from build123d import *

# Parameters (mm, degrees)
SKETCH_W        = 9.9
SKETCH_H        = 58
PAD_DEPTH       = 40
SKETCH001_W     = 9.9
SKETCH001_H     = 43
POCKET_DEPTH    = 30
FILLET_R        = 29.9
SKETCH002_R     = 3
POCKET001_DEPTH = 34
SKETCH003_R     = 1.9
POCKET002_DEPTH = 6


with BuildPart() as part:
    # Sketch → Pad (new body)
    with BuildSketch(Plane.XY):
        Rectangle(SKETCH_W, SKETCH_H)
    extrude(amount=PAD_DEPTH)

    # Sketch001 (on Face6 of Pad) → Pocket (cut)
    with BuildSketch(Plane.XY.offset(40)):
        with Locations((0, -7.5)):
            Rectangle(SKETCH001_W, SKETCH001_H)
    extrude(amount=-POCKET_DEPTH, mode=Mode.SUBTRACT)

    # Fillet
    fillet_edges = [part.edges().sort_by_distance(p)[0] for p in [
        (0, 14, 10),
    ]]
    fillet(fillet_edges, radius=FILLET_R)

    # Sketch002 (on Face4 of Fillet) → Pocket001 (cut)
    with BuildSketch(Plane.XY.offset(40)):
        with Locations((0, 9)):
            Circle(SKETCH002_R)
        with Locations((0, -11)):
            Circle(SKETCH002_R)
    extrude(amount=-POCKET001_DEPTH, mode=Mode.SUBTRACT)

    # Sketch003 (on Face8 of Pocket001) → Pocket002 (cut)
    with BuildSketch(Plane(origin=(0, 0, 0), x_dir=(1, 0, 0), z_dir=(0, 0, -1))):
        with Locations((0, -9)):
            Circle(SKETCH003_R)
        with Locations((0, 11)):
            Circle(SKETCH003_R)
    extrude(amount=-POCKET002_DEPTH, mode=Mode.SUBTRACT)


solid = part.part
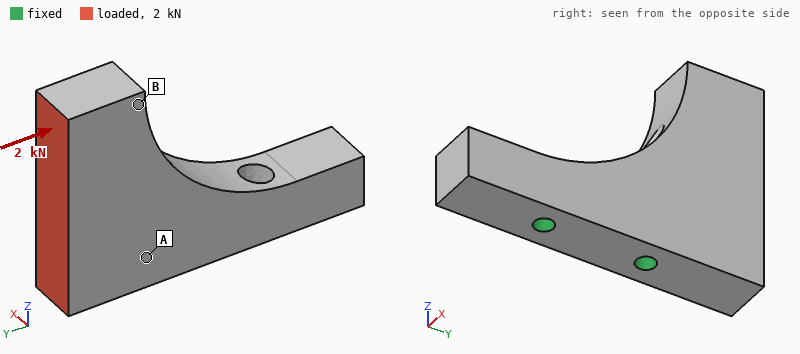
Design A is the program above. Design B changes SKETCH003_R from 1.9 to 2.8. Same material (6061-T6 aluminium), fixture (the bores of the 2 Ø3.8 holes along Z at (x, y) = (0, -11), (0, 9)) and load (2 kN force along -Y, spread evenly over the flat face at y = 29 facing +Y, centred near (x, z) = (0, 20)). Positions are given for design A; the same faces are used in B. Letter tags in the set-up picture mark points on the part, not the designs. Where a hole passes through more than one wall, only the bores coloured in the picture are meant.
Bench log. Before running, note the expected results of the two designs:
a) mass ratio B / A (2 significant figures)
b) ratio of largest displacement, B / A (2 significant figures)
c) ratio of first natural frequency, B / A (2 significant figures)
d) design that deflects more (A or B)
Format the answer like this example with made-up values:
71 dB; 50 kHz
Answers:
0.99; 0.88; 1.1; A
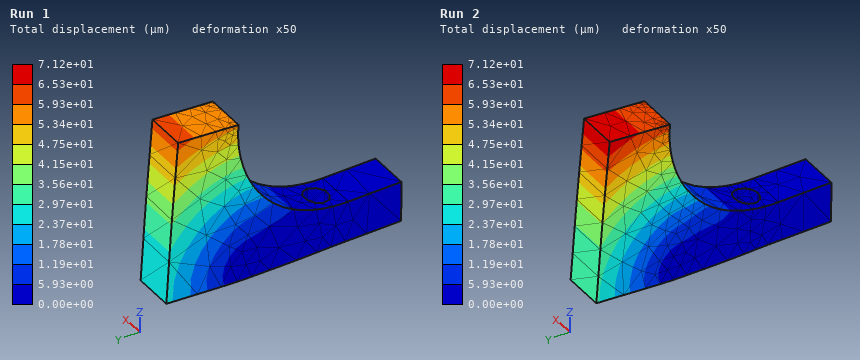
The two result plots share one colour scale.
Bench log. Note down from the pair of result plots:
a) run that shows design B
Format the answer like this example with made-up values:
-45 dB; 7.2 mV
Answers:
Run 1
